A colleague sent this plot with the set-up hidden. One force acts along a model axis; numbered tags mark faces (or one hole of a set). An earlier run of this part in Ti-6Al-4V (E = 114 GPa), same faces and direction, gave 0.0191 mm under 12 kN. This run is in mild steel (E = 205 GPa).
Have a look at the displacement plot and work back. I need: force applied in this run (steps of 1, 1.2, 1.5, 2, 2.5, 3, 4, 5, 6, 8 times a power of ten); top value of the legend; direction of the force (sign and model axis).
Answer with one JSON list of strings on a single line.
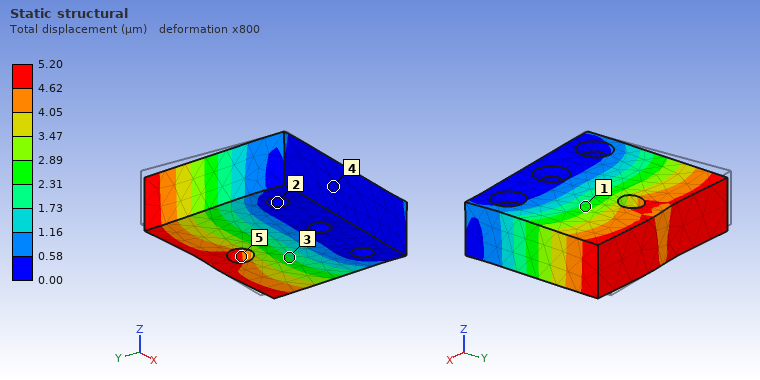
["6 kN", "5.20 µm", "+X"]
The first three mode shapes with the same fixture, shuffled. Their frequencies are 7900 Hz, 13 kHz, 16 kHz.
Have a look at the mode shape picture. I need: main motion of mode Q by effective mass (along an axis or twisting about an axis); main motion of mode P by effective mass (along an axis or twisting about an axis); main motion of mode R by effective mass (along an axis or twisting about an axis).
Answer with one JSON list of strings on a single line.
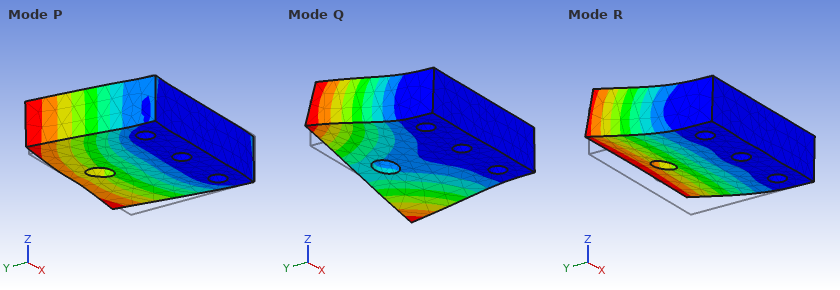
["twisting about Y", "along X", "along Z"]
